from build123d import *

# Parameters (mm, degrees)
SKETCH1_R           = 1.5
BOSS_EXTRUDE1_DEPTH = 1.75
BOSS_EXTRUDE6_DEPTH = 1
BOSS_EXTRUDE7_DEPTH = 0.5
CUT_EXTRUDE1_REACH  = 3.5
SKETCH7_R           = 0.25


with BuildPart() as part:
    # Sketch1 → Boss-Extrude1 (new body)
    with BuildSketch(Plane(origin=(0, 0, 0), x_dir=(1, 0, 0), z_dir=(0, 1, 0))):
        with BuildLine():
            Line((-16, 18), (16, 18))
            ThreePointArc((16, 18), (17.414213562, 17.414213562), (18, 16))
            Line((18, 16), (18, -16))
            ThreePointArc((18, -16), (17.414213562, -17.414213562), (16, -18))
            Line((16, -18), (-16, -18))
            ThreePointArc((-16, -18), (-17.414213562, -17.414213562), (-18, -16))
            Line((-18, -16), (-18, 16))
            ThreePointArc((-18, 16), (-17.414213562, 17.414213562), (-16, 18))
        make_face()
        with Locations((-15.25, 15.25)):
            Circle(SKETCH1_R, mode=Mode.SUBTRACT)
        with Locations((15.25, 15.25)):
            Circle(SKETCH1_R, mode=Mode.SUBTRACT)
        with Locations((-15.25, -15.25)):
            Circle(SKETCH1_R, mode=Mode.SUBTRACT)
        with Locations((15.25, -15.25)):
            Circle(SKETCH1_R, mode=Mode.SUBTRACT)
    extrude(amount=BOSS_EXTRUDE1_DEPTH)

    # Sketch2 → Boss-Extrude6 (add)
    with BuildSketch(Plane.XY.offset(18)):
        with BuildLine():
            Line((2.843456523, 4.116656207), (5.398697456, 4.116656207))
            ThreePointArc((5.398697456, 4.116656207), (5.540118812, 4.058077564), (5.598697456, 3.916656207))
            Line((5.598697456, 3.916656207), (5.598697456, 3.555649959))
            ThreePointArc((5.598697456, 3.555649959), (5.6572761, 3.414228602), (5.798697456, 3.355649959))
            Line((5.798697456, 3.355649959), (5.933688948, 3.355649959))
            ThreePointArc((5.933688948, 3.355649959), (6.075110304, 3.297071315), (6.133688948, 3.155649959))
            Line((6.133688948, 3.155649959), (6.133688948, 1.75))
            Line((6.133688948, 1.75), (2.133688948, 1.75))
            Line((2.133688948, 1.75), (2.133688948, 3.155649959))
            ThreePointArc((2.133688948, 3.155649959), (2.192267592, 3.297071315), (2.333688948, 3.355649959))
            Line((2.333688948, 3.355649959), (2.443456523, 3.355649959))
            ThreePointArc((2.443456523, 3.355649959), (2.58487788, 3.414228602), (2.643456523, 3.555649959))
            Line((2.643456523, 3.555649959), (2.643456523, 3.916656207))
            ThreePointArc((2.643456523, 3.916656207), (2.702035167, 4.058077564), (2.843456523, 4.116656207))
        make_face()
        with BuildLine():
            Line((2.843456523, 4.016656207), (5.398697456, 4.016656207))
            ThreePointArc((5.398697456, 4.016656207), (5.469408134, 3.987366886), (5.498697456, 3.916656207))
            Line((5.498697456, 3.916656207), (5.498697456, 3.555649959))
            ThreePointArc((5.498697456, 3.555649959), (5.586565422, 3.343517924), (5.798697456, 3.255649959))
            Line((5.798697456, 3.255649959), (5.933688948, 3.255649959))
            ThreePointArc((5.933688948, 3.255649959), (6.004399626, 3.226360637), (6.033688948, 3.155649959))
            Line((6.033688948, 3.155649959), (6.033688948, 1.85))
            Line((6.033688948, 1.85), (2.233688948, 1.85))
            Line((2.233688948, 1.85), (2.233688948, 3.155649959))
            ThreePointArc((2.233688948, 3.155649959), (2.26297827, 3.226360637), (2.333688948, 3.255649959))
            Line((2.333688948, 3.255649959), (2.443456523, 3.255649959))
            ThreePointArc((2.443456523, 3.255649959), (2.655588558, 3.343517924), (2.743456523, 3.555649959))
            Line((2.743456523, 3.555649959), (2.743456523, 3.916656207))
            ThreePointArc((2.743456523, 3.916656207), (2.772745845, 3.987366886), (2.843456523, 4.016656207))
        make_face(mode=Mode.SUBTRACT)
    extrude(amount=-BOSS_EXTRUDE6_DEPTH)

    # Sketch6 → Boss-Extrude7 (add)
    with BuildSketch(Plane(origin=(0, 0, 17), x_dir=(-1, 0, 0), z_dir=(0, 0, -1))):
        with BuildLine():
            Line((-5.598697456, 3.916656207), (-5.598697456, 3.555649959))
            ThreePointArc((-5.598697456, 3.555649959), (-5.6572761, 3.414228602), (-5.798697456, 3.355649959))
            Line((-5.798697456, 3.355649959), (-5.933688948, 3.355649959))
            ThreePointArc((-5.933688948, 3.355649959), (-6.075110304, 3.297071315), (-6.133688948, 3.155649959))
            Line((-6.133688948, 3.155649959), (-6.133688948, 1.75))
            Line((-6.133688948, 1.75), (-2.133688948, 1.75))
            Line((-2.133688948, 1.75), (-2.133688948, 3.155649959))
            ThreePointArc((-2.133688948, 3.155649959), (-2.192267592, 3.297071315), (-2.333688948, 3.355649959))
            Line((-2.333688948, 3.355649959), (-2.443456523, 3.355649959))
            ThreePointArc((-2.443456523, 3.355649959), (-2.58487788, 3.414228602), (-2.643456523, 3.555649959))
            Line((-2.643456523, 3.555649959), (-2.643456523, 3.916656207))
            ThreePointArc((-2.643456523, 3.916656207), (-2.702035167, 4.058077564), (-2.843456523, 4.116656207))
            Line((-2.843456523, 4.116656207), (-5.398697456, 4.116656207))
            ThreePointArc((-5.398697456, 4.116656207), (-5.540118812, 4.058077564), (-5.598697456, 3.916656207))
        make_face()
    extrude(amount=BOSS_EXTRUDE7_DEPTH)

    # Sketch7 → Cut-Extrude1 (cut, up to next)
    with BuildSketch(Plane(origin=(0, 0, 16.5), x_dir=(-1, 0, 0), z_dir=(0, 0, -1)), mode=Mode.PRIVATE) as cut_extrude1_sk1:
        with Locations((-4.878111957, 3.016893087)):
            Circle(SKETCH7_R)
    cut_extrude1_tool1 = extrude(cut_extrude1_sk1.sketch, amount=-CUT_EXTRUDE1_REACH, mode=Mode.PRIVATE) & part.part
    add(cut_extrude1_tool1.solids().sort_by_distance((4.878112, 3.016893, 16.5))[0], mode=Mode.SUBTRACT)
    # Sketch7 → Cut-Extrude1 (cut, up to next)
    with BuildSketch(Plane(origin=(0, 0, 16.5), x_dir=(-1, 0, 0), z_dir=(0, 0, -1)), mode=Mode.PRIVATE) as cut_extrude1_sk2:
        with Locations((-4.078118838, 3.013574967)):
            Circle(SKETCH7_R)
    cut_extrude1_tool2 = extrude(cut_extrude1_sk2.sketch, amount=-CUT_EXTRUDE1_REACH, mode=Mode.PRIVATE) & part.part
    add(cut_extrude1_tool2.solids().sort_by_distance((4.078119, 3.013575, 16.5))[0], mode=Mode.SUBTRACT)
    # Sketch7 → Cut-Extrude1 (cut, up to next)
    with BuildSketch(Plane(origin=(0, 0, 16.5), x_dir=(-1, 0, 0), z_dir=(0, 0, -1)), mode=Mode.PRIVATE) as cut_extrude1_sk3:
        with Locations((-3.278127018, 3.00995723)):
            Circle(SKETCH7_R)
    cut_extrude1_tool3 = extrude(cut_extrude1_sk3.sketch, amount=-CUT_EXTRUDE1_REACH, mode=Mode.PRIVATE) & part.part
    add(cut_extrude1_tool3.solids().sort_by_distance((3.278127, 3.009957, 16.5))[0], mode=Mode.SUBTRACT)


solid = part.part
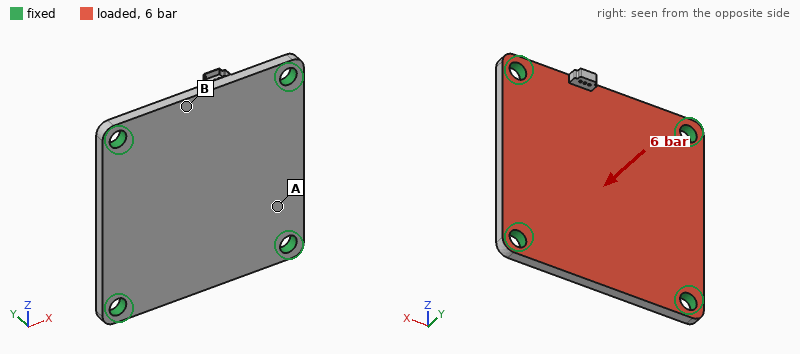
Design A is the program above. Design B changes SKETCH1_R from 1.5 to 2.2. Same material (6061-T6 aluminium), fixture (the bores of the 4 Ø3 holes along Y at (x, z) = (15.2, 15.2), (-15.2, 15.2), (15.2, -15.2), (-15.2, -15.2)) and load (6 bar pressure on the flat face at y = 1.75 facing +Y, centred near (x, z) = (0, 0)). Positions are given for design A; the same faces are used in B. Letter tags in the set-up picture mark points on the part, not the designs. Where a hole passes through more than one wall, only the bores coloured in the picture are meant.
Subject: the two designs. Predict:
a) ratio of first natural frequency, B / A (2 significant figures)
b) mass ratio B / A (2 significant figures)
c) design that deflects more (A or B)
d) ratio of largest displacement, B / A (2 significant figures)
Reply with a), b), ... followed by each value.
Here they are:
a) 1.1
b) 0.97
c) A
d) 0.82
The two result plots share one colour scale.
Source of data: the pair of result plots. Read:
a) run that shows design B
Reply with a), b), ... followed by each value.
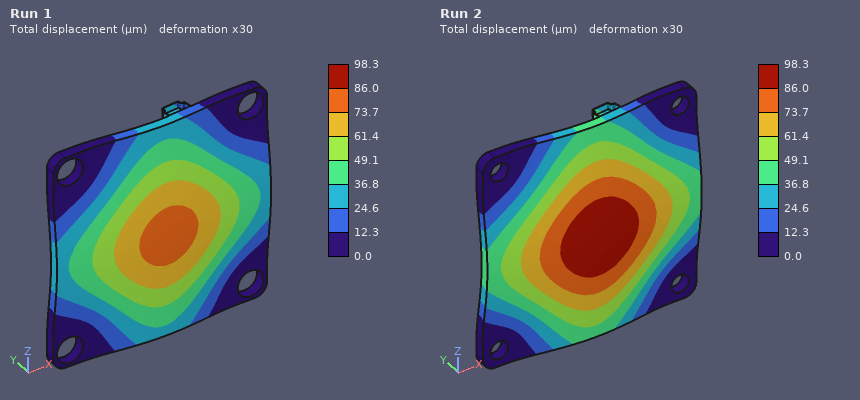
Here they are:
a) Run 1
